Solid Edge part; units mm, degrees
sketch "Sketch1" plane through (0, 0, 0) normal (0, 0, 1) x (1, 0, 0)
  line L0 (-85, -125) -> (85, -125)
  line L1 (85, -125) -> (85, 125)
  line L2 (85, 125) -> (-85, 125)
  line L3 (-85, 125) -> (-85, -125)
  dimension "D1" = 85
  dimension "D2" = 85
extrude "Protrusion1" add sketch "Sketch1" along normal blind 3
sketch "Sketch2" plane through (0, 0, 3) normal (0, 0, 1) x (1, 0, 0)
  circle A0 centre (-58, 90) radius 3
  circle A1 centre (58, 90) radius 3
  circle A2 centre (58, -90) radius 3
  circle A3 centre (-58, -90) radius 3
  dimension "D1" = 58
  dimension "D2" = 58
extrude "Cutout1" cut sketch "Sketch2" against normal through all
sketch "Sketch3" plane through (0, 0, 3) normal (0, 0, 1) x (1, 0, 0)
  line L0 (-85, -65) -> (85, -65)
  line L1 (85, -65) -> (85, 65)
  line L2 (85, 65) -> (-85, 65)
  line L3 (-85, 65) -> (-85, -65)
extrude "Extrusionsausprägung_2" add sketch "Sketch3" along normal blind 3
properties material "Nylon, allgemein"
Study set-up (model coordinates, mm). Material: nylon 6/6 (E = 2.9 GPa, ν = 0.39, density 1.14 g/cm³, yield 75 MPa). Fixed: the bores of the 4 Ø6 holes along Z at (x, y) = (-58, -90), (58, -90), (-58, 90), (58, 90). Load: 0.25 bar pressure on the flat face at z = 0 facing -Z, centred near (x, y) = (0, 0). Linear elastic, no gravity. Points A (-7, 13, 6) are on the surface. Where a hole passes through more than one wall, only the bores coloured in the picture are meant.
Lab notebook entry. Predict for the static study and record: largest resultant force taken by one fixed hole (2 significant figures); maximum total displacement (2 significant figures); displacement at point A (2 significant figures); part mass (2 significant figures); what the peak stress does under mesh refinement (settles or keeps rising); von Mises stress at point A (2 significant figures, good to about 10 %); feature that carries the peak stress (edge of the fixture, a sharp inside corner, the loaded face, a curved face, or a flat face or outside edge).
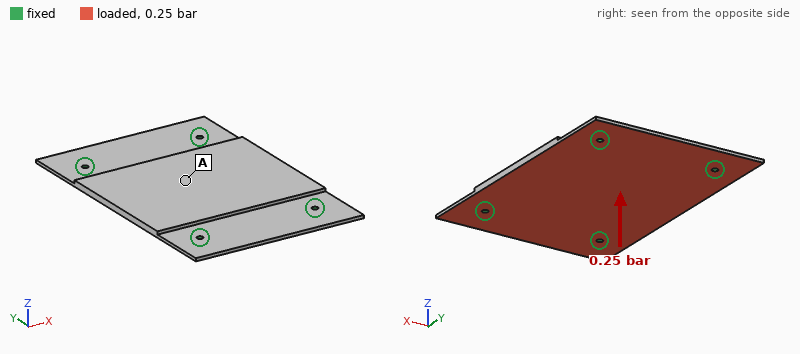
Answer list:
590 N
3.5 mm
3.5 mm
220 g
keeps rising
7.9 MPa
edge of the fixture
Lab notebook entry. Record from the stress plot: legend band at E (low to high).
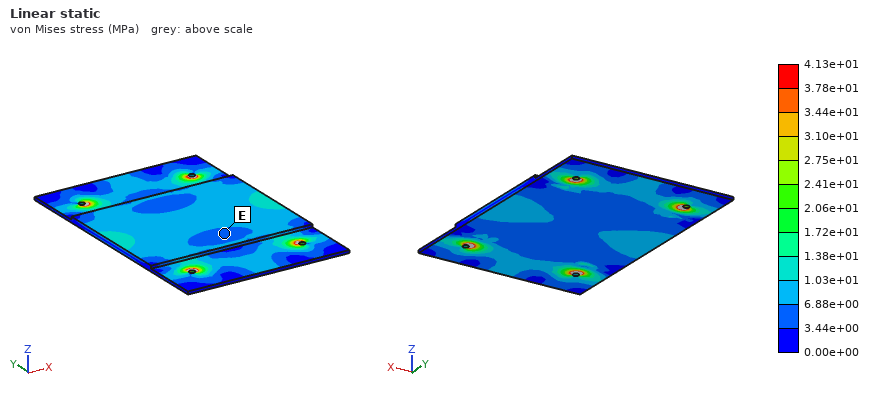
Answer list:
3.44e+00 to 6.88e+00 MPa
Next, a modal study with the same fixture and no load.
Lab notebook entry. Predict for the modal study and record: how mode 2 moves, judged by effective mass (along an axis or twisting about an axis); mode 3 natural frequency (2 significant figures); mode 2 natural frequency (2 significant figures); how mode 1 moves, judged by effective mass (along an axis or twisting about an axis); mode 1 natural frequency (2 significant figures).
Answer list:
twisting about Y
340 Hz
240 Hz
along Z
180 Hz
